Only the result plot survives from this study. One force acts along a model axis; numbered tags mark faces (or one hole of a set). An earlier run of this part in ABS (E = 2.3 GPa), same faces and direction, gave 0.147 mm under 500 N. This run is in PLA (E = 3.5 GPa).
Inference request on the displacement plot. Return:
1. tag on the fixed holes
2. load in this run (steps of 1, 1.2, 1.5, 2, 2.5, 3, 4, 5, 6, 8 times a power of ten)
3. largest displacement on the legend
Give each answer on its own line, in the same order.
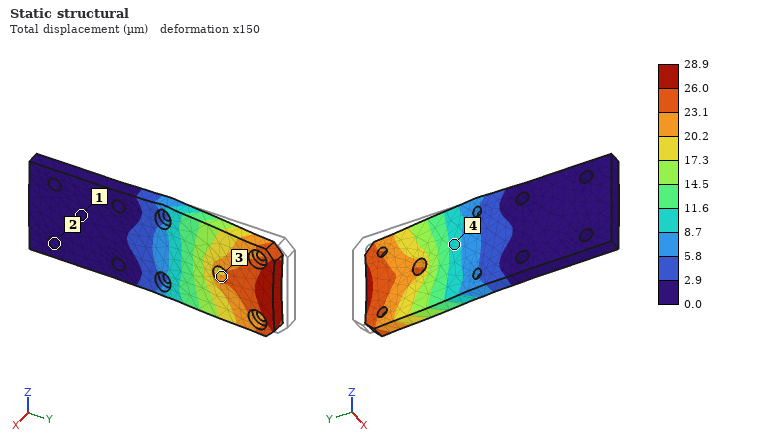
2
150 N
28.9 µm
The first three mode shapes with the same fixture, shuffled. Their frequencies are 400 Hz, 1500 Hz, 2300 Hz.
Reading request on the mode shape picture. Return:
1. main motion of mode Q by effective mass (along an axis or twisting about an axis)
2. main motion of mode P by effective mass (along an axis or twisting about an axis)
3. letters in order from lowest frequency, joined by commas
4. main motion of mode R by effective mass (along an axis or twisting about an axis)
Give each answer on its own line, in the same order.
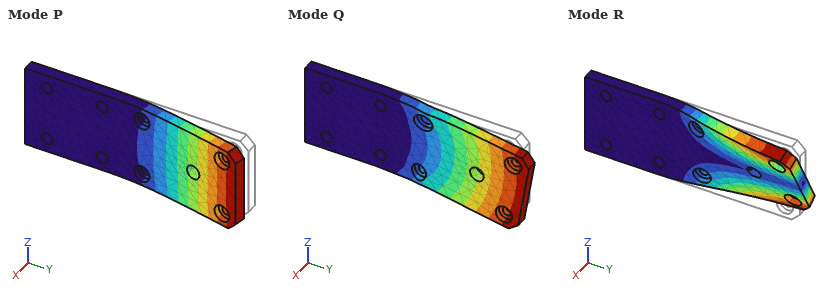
along Z
along X
P, R, Q
twisting about Y
